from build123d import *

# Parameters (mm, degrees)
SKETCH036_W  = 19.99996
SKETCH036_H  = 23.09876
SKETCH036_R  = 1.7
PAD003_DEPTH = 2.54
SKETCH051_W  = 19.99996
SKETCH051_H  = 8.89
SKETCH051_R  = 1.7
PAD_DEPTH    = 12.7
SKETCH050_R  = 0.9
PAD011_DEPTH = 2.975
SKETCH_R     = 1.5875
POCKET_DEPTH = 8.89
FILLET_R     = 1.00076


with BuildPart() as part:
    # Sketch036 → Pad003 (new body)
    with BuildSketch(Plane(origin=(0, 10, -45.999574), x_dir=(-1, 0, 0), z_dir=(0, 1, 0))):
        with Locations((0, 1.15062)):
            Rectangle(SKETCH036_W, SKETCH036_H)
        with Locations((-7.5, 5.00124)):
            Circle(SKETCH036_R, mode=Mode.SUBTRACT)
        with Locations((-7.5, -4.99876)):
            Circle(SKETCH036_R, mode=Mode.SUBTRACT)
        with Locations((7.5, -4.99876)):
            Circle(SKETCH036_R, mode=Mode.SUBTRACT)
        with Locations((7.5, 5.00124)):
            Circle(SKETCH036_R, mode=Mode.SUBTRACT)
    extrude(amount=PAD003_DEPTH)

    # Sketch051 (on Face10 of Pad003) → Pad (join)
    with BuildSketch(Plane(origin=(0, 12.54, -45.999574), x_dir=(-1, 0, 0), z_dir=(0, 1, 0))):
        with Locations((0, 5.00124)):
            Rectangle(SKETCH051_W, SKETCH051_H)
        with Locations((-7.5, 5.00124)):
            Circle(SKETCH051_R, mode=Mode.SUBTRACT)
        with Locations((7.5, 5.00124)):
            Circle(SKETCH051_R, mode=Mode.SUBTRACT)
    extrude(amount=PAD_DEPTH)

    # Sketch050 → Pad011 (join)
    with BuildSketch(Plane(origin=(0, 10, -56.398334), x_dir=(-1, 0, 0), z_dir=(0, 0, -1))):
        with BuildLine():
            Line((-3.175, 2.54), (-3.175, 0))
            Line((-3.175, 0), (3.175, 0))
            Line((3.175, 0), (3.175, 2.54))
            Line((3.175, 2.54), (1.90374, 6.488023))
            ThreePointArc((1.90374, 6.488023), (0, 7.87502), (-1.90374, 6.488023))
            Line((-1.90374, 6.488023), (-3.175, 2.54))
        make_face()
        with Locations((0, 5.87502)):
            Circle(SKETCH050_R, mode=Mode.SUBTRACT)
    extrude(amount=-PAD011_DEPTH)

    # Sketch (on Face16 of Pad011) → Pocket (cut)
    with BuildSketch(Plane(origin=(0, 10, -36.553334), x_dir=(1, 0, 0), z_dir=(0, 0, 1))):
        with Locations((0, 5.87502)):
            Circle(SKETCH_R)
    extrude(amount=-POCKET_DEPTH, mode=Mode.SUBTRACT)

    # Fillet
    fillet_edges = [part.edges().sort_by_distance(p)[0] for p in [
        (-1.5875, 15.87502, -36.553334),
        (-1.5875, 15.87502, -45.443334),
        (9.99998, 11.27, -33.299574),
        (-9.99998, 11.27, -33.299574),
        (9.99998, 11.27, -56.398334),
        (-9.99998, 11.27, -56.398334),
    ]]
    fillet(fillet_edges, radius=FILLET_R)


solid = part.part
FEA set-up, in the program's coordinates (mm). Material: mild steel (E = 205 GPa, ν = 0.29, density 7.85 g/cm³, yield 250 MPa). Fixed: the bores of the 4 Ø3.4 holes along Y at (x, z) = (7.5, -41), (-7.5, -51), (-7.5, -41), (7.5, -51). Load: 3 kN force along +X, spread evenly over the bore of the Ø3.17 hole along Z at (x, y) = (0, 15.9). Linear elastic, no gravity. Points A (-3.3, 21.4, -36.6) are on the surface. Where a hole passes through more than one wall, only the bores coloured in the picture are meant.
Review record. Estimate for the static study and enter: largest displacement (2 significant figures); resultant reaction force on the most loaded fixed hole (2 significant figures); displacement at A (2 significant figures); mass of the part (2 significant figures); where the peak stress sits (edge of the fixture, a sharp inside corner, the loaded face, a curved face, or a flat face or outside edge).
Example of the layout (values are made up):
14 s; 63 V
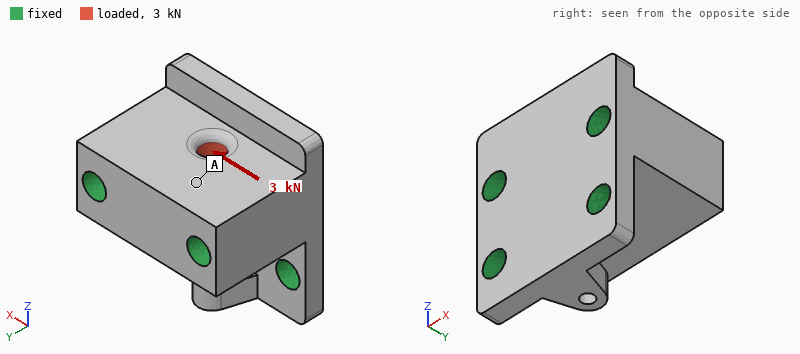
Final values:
0.85 µm; 1.5 kN; 0.16 µm; 24 g; the loaded face
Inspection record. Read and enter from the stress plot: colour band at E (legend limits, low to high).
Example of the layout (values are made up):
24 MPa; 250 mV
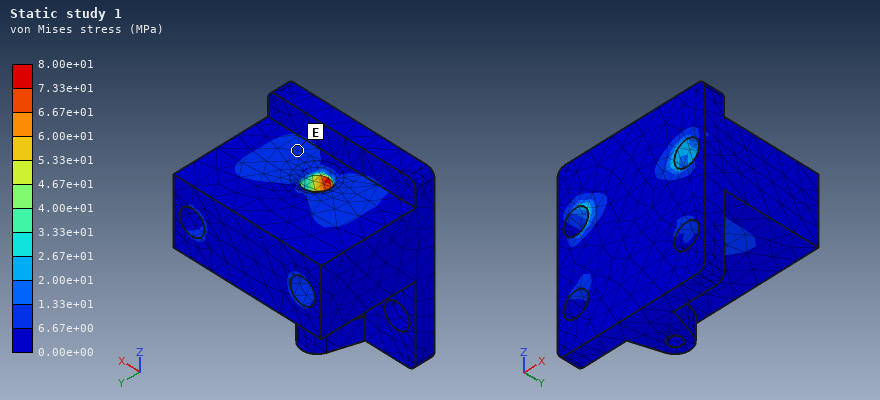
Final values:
6.67e+00 to 1.33e+01 MPa
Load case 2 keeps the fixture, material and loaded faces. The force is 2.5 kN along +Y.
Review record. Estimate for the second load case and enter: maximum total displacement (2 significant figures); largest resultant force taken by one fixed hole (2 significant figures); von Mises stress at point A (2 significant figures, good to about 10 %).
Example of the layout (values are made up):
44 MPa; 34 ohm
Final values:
1.2 µm; 1.2 kN; 13 MPa
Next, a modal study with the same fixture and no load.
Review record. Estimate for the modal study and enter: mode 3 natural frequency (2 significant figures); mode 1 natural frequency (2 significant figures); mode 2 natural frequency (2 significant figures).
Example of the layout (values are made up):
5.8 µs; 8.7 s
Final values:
70 kHz; 38 kHz; 63 kHz
